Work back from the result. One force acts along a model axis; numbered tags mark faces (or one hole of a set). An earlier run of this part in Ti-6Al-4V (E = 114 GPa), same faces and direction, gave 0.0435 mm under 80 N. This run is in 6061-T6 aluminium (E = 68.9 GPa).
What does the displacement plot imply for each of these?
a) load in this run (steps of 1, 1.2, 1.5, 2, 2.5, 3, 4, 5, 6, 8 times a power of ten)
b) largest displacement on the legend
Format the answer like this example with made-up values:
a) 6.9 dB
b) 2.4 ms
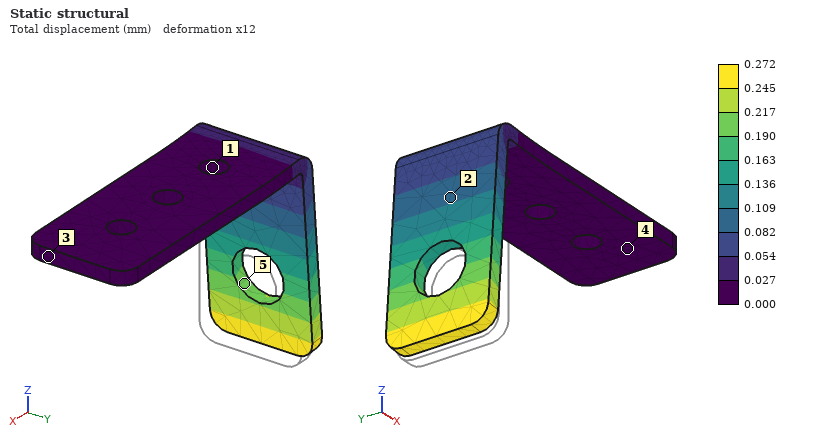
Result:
a) 300 N
b) 0.272 mm
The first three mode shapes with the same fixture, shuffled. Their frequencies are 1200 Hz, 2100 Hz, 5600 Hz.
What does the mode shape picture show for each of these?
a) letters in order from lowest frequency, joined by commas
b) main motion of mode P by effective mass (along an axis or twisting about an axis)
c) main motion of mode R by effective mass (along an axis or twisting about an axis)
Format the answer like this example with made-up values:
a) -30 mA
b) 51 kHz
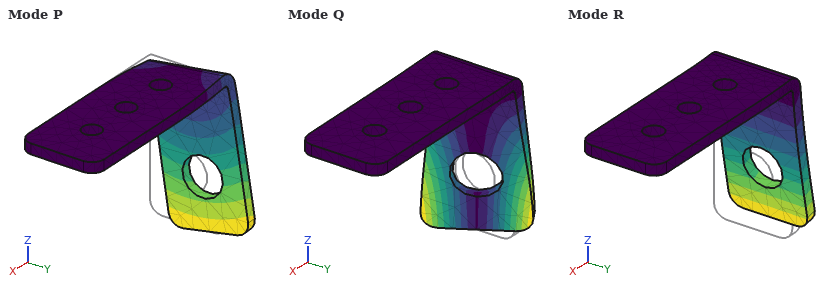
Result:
a) R, P, Q
b) along Y
c) along X
